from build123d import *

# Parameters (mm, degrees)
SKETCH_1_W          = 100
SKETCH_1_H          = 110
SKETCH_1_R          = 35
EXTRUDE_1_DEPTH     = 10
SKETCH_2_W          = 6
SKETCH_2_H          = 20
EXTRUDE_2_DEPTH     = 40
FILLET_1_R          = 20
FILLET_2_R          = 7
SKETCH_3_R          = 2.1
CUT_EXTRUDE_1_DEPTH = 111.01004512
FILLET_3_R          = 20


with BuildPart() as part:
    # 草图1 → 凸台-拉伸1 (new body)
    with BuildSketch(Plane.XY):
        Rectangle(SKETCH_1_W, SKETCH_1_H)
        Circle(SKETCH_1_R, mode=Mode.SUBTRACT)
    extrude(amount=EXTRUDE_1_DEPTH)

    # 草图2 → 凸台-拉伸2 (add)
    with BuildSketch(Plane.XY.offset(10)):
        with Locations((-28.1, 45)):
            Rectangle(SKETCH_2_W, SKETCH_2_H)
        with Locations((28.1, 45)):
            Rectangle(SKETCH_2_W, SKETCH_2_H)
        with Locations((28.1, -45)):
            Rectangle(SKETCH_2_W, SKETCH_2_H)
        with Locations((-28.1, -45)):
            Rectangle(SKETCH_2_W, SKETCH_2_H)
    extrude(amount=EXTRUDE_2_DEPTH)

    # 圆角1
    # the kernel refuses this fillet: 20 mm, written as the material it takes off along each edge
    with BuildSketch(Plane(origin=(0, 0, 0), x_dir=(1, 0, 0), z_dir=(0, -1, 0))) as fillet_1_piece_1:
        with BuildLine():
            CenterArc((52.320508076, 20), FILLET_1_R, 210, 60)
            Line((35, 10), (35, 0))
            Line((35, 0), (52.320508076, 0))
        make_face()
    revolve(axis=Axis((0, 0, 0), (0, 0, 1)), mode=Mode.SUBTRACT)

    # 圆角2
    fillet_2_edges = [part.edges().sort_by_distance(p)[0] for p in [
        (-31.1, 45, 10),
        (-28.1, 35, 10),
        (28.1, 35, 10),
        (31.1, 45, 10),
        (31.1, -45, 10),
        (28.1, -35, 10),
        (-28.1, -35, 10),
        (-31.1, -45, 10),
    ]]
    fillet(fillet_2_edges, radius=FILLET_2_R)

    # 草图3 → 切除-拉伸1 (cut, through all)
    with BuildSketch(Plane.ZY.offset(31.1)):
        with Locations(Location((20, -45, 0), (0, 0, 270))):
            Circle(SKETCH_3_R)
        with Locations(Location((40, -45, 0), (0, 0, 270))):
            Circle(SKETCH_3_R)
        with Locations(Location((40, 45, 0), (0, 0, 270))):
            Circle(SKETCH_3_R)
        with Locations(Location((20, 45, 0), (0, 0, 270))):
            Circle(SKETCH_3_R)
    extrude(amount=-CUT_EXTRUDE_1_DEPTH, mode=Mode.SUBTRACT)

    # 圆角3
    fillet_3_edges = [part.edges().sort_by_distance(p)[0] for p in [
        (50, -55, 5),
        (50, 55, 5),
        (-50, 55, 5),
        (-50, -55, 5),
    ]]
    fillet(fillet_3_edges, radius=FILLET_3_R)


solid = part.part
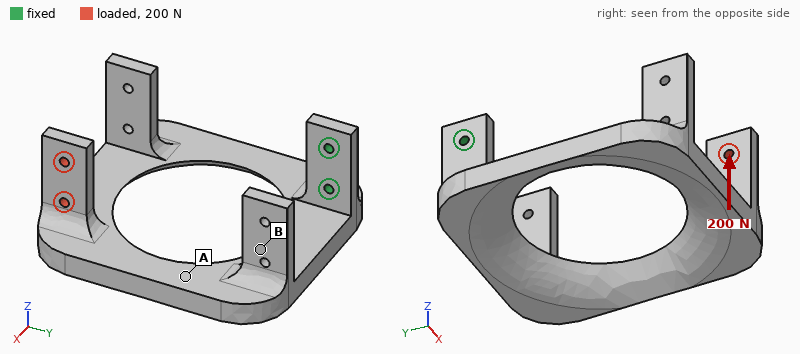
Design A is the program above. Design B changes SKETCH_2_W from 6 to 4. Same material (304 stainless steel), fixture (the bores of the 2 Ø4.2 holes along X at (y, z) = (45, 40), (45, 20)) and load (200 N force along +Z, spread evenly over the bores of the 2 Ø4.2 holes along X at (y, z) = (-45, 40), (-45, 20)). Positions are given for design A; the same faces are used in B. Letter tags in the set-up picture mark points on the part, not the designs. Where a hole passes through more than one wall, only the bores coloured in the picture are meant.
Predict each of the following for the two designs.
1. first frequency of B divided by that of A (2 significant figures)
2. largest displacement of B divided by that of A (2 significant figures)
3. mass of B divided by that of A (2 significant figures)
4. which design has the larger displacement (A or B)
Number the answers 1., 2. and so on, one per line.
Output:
1. 0.81
2. 1.4
3. 0.92
4. B
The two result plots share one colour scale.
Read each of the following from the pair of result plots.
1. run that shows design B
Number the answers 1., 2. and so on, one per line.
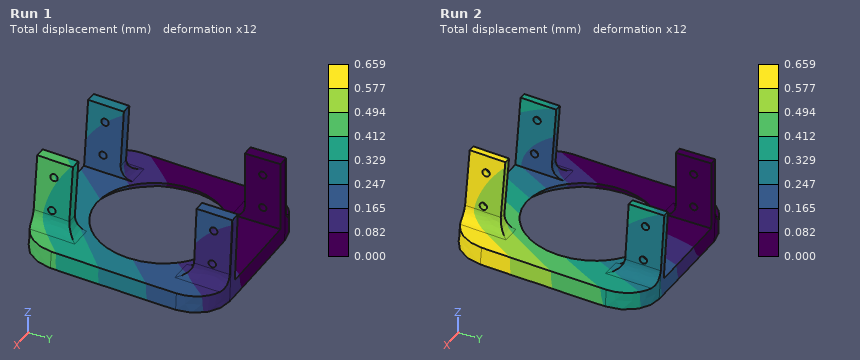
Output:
1. Run 2
